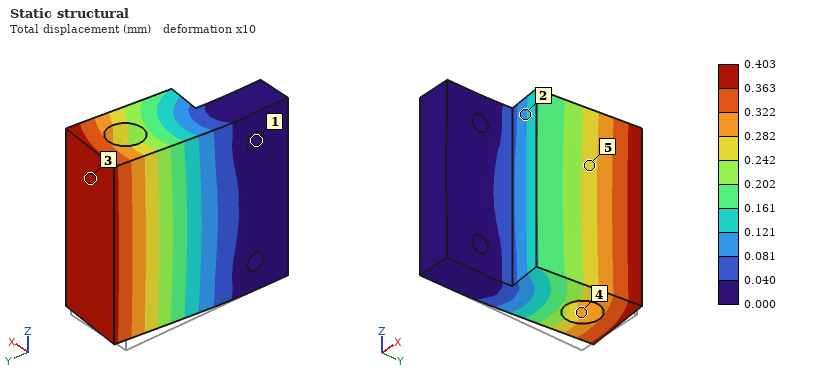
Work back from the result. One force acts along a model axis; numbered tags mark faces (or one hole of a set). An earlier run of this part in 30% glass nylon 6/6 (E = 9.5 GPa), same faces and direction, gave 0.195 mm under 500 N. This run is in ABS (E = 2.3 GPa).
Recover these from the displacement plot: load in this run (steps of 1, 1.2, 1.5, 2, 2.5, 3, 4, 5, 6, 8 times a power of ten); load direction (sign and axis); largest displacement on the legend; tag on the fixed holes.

250 N
+X
0.403 mm
1
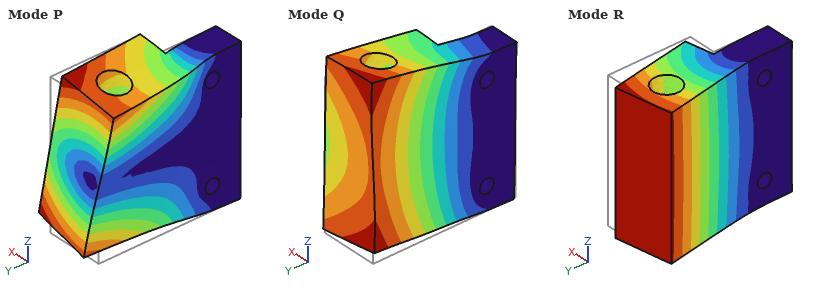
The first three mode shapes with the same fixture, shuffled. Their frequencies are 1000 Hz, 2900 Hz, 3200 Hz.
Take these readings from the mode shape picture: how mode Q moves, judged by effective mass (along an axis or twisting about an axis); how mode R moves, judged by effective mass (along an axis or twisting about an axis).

along Z
along X
